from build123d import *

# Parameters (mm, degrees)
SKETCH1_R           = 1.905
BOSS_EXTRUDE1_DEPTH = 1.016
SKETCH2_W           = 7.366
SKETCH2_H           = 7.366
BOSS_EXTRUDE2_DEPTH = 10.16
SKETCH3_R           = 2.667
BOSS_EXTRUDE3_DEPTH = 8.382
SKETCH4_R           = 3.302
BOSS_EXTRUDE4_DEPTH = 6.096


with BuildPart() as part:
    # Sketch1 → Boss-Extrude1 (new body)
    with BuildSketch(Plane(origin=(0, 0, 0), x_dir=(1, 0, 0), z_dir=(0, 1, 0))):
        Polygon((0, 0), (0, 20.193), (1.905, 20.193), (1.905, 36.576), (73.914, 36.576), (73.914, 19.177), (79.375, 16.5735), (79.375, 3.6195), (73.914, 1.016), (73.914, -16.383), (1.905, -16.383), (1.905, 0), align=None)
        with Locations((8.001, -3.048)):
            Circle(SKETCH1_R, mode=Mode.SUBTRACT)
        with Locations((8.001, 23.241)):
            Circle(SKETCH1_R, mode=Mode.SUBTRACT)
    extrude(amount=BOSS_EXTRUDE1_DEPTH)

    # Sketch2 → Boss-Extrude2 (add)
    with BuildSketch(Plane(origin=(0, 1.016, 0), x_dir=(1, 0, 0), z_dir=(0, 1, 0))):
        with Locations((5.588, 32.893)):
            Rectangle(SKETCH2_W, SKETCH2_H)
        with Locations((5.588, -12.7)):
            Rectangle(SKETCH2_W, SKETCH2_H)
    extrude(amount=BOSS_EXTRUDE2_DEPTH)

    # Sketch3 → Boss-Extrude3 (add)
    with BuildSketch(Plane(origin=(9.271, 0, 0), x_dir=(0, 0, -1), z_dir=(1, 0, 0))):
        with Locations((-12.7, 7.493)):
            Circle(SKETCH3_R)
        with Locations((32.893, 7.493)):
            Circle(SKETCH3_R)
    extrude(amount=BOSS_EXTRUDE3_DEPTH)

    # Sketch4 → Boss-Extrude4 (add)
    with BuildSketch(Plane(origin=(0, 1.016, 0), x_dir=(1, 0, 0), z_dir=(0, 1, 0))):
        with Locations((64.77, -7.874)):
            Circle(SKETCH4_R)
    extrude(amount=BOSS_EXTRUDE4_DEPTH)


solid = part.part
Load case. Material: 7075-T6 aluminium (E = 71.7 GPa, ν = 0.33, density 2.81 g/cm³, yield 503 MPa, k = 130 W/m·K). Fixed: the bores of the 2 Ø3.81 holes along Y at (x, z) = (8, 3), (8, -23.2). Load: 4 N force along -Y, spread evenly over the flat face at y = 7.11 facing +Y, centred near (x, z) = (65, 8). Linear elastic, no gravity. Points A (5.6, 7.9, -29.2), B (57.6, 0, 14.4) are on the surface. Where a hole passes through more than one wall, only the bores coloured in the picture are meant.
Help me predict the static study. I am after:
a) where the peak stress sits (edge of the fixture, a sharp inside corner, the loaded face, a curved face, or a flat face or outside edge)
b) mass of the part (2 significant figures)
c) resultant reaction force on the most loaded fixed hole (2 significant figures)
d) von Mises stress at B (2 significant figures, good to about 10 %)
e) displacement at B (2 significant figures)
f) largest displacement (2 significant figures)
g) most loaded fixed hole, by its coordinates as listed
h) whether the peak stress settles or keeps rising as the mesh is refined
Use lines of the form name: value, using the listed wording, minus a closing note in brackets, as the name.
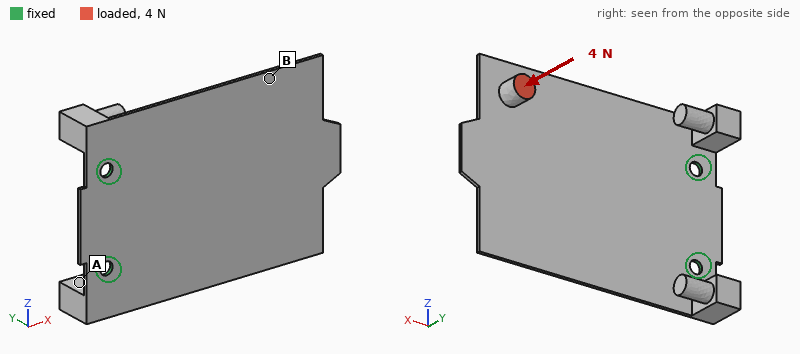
where the peak stress sits: edge of the fixture
mass of the part: 16 g
resultant reaction force on the most loaded fixed hole: 4.0 N
von Mises stress at B: 5.9 MPa
displacement at B: 0.68 mm
largest displacement: 1.0 mm
most loaded fixed hole, by its coordinates as listed: (8, 3)
whether the peak stress settles or keeps rising as the mesh is refined: keeps rising
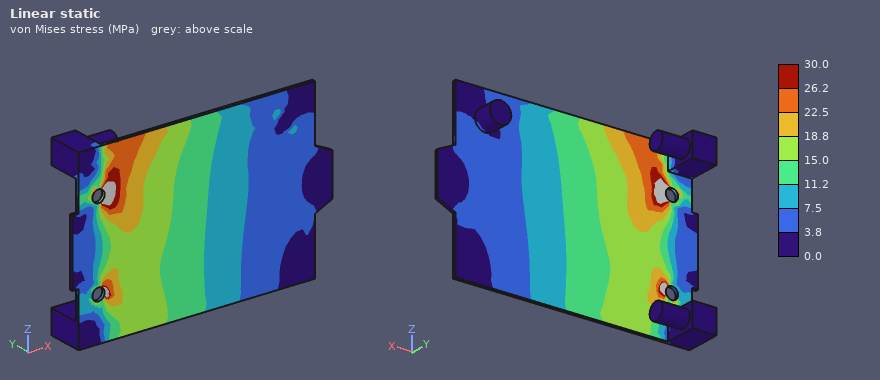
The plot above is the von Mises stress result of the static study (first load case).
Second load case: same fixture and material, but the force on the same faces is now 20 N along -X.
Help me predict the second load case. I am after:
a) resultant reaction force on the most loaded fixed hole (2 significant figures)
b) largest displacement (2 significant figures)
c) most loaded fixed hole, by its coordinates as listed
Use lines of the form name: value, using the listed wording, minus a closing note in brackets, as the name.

resultant reaction force on the most loaded fixed hole: 23 N
largest displacement: 0.96 mm
most loaded fixed hole, by its coordinates as listed: (8, 3)
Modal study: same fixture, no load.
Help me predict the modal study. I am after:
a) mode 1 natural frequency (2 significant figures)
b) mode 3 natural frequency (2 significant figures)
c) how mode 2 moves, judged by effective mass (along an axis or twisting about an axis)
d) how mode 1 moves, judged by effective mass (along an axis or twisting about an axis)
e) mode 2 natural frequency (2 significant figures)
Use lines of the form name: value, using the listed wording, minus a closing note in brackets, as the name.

mode 1 natural frequency: 170 Hz
mode 3 natural frequency: 1100 Hz
how mode 2 moves, judged by effective mass: twisting about X
how mode 1 moves, judged by effective mass: along Y
mode 2 natural frequency: 520 Hz
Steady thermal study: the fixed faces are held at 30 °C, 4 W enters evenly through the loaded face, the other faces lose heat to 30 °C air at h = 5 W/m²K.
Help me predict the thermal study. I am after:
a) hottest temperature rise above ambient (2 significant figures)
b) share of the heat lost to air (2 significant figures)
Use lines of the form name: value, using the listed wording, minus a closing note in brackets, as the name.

hottest temperature rise above ambient: 46 K
share of the heat lost to air: 17 %
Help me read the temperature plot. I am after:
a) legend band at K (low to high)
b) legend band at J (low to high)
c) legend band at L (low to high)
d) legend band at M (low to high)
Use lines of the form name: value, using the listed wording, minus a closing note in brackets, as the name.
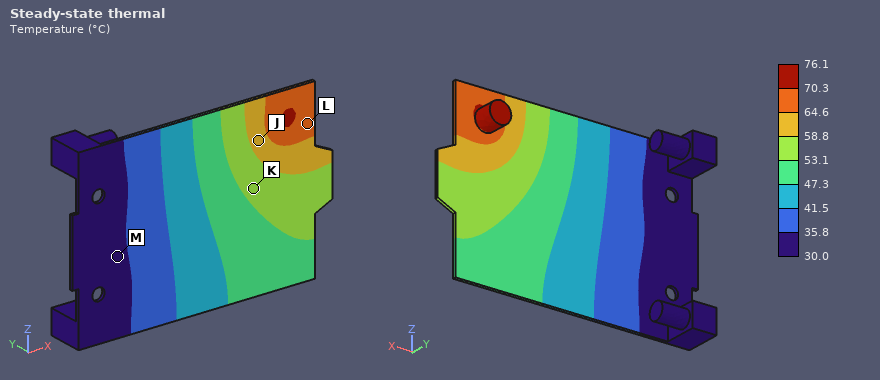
legend band at K: 53.1 to 58.8 °C
legend band at J: 58.8 to 64.6 °C
legend band at L: 64.6 to 70.3 °C
legend band at M: 30.0 to 35.8 °C
